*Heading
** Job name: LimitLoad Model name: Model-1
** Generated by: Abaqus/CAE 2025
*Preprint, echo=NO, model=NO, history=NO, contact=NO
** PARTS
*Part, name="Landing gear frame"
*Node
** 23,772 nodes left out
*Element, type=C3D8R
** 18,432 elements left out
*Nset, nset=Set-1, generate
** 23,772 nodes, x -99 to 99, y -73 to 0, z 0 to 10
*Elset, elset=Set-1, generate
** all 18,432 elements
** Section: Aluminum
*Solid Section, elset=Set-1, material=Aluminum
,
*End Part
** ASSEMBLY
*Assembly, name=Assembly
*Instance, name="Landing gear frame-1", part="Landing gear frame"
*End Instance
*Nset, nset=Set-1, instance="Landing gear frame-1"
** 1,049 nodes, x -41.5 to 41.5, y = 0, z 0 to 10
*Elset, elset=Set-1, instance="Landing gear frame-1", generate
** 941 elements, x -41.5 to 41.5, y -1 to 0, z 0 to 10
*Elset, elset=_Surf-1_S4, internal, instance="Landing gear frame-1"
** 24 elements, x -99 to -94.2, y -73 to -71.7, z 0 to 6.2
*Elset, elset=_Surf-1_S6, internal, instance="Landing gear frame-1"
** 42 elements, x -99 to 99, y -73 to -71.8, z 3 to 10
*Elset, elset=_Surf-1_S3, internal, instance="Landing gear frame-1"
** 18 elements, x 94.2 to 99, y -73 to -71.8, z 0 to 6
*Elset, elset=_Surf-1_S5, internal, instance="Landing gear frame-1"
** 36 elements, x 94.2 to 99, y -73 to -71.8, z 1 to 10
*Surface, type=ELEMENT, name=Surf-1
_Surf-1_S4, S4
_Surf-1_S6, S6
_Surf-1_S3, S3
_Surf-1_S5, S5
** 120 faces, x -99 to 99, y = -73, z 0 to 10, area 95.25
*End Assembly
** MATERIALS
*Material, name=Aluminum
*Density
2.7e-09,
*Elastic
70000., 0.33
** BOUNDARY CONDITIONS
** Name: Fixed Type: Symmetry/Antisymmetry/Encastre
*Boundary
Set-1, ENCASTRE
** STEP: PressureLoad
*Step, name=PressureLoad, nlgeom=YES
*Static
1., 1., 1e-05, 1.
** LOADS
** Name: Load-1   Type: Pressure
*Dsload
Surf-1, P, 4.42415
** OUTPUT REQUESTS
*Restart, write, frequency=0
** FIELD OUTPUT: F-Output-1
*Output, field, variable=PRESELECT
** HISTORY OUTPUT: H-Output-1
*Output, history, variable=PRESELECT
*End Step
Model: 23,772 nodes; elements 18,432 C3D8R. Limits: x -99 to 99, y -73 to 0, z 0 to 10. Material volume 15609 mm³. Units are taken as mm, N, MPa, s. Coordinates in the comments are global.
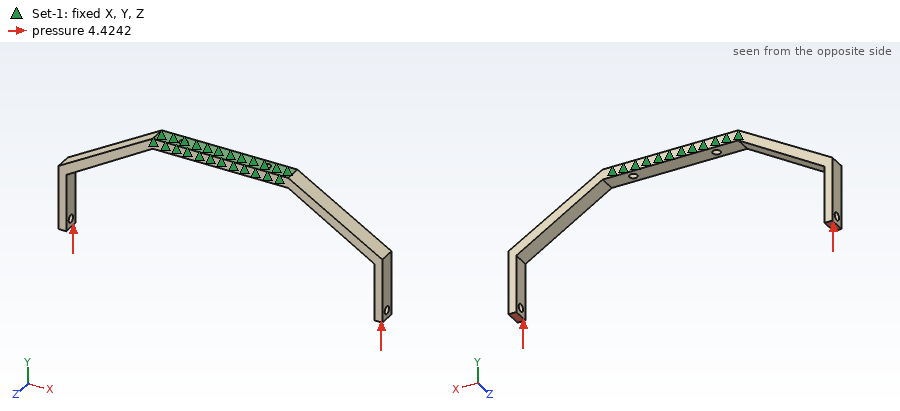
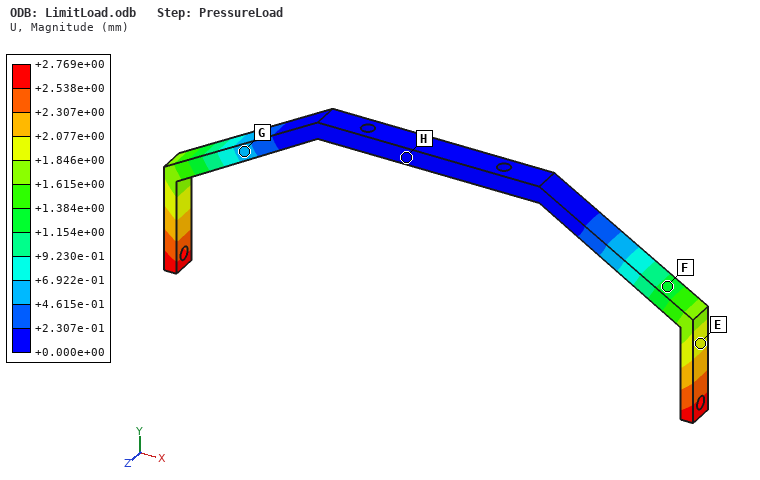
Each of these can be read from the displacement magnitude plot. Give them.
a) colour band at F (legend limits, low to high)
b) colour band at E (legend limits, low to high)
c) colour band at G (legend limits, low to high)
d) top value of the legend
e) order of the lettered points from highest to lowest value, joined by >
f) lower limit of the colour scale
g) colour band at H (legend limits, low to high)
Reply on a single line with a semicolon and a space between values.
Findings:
+1.154e+00 to +1.384e+00 mm; +1.846e+00 to +2.077e+00 mm; +4.615e-01 to +6.922e-01 mm; +2.769e+00 mm; E > F > G > H; +0.000e+00 mm; +0.000e+00 to +2.307e-01 mm
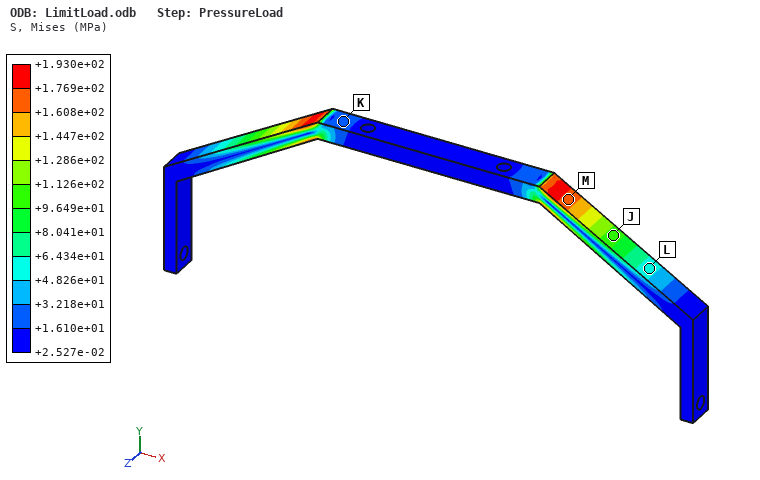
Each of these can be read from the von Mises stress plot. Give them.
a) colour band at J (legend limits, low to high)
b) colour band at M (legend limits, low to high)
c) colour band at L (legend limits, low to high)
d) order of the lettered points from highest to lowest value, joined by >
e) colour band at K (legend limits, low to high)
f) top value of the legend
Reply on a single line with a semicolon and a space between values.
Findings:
+9.649e+01 to +1.126e+02 MPa; +1.608e+02 to +1.769e+02 MPa; +4.826e+01 to +6.434e+01 MPa; M > J > L > K; +1.610e+01 to +3.218e+01 MPa; +1.930e+02 MPa
